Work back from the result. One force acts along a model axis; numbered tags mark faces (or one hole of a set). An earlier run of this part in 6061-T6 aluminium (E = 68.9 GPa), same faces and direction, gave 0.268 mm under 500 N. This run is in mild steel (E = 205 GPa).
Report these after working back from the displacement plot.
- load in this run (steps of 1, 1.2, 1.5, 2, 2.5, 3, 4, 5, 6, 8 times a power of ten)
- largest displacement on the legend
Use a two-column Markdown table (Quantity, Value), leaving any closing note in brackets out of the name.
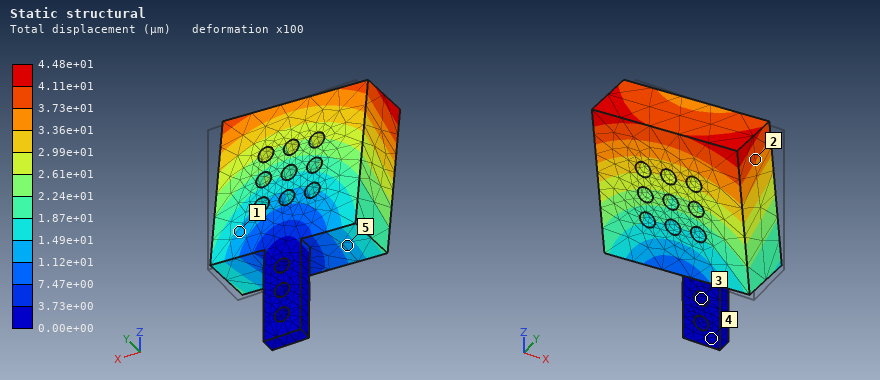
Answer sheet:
| Quantity | Value |
|---|---|
| load in this run | 250 N |
| largest displacement on the legend | 4.48e+01 µm |
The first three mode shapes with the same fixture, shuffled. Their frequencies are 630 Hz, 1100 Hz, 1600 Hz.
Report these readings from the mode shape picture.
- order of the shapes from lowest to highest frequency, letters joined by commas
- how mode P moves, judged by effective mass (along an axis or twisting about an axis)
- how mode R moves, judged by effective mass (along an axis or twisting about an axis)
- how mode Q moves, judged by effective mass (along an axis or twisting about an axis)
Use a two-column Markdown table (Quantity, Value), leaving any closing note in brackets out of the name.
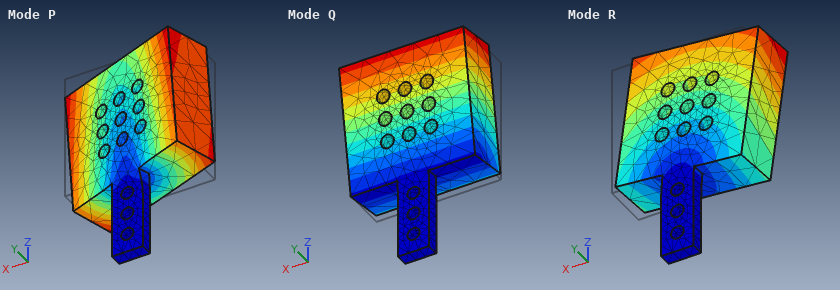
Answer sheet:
| Quantity | Value |
|---|---|
| order of the shapes from lowest to highest frequency, letters joined by commas | Q, R, P |
| how mode P moves, judged by effective mass | twisting about Z |
| how mode R moves, judged by effective mass | along X |
| how mode Q moves, judged by effective mass | along Y |
